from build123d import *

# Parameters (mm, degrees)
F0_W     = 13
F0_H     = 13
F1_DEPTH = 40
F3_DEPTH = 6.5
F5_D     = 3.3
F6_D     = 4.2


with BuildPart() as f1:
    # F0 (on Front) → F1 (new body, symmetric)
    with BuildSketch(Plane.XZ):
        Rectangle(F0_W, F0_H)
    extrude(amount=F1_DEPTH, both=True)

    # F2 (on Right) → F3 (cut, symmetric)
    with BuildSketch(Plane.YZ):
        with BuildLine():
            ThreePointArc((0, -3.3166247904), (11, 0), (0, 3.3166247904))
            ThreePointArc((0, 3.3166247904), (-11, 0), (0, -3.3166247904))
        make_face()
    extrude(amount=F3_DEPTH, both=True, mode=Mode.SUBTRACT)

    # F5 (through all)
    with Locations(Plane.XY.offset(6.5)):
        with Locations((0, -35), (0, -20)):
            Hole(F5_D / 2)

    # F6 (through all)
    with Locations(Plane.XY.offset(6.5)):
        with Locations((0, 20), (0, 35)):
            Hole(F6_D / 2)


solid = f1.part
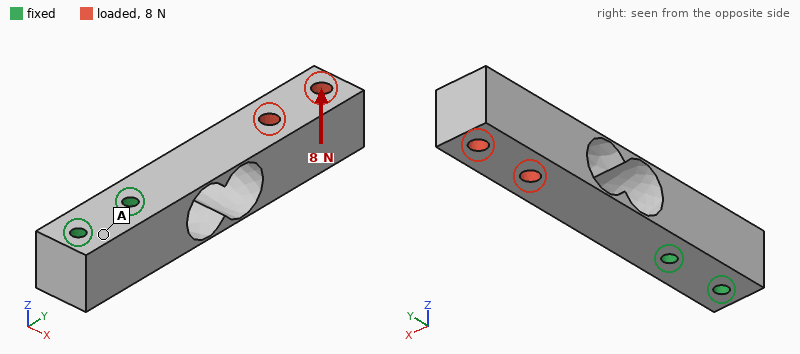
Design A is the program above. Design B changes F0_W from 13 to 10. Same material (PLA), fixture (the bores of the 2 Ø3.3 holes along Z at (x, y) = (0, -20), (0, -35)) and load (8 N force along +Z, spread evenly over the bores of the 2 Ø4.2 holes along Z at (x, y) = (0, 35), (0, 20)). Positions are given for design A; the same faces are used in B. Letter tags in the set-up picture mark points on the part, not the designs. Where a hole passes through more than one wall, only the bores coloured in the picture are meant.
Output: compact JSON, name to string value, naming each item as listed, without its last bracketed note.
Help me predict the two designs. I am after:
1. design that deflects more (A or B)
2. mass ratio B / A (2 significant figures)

{"design that deflects more": "B", "mass ratio B / A": "0.76"}
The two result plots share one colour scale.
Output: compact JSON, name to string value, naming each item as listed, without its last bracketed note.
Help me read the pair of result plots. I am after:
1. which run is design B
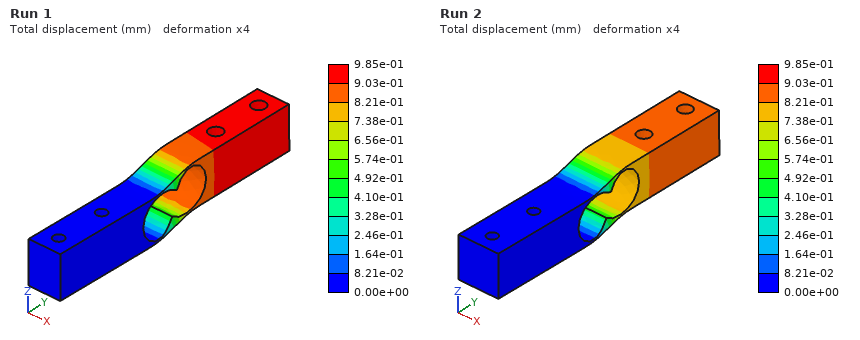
{"which run is design B": "Run 1"}
